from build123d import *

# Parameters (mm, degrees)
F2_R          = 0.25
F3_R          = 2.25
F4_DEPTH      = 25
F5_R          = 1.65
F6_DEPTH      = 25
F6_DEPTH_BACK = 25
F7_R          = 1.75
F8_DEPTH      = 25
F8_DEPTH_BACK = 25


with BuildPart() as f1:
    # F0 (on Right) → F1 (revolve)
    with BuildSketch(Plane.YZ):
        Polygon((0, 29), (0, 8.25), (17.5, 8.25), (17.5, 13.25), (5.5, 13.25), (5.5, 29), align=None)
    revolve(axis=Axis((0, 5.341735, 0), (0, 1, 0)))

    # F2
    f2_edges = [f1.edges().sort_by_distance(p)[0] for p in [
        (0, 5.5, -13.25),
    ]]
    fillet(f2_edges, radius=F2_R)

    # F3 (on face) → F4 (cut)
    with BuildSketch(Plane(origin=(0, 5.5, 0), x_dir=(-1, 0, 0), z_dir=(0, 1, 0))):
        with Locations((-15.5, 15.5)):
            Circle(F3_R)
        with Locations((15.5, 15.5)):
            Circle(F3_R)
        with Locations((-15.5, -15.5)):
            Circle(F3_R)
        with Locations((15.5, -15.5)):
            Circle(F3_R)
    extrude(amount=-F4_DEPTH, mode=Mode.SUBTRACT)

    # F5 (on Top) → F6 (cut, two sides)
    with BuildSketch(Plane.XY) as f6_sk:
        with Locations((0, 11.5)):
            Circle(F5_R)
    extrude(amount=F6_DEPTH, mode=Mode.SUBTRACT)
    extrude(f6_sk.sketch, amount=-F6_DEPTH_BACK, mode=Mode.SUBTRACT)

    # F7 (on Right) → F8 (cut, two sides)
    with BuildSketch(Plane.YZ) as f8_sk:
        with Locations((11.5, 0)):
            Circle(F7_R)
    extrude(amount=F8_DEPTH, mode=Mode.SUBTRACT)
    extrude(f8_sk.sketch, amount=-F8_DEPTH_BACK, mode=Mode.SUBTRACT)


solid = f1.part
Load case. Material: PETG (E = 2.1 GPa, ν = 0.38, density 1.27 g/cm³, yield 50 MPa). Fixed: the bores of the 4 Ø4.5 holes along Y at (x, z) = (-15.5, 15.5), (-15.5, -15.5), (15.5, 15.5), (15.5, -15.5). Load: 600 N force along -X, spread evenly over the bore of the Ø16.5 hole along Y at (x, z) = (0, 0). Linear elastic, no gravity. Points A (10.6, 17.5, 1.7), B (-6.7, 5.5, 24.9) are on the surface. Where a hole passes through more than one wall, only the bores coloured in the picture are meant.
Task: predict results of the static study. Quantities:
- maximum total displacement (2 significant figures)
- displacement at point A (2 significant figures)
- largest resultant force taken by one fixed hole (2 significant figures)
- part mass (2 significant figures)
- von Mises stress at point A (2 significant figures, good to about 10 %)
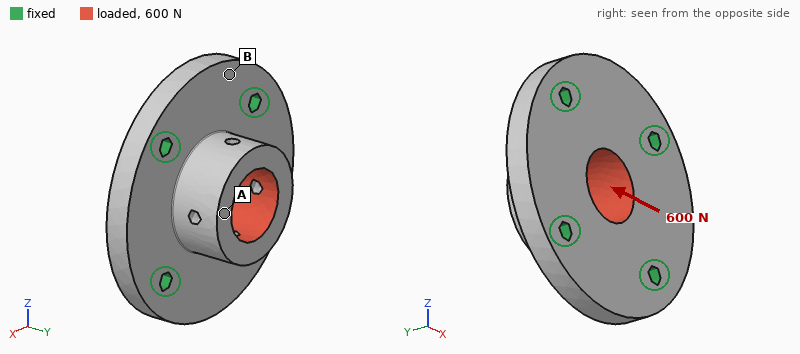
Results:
69 µm
66 µm
170 N
21 g
1.8 MPa
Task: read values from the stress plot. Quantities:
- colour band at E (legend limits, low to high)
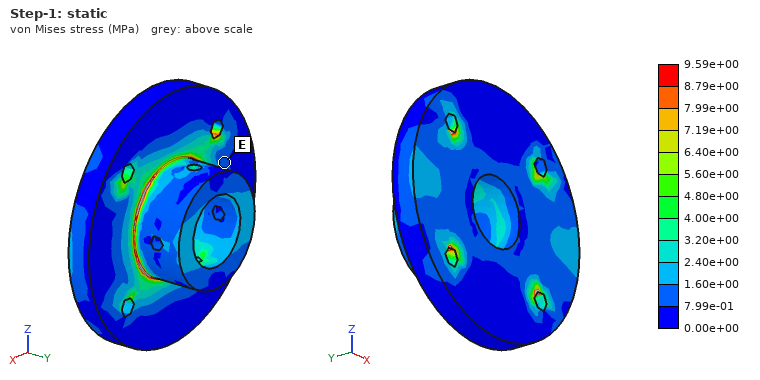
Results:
7.99e-01 to 1.60e+00 MPa
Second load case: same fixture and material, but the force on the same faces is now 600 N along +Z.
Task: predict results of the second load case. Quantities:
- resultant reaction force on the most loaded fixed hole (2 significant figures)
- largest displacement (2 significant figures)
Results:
170 N
69 µm
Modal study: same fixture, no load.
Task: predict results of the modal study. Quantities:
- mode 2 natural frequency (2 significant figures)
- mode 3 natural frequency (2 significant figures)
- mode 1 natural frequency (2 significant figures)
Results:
4900 Hz
5000 Hz
4900 Hz
